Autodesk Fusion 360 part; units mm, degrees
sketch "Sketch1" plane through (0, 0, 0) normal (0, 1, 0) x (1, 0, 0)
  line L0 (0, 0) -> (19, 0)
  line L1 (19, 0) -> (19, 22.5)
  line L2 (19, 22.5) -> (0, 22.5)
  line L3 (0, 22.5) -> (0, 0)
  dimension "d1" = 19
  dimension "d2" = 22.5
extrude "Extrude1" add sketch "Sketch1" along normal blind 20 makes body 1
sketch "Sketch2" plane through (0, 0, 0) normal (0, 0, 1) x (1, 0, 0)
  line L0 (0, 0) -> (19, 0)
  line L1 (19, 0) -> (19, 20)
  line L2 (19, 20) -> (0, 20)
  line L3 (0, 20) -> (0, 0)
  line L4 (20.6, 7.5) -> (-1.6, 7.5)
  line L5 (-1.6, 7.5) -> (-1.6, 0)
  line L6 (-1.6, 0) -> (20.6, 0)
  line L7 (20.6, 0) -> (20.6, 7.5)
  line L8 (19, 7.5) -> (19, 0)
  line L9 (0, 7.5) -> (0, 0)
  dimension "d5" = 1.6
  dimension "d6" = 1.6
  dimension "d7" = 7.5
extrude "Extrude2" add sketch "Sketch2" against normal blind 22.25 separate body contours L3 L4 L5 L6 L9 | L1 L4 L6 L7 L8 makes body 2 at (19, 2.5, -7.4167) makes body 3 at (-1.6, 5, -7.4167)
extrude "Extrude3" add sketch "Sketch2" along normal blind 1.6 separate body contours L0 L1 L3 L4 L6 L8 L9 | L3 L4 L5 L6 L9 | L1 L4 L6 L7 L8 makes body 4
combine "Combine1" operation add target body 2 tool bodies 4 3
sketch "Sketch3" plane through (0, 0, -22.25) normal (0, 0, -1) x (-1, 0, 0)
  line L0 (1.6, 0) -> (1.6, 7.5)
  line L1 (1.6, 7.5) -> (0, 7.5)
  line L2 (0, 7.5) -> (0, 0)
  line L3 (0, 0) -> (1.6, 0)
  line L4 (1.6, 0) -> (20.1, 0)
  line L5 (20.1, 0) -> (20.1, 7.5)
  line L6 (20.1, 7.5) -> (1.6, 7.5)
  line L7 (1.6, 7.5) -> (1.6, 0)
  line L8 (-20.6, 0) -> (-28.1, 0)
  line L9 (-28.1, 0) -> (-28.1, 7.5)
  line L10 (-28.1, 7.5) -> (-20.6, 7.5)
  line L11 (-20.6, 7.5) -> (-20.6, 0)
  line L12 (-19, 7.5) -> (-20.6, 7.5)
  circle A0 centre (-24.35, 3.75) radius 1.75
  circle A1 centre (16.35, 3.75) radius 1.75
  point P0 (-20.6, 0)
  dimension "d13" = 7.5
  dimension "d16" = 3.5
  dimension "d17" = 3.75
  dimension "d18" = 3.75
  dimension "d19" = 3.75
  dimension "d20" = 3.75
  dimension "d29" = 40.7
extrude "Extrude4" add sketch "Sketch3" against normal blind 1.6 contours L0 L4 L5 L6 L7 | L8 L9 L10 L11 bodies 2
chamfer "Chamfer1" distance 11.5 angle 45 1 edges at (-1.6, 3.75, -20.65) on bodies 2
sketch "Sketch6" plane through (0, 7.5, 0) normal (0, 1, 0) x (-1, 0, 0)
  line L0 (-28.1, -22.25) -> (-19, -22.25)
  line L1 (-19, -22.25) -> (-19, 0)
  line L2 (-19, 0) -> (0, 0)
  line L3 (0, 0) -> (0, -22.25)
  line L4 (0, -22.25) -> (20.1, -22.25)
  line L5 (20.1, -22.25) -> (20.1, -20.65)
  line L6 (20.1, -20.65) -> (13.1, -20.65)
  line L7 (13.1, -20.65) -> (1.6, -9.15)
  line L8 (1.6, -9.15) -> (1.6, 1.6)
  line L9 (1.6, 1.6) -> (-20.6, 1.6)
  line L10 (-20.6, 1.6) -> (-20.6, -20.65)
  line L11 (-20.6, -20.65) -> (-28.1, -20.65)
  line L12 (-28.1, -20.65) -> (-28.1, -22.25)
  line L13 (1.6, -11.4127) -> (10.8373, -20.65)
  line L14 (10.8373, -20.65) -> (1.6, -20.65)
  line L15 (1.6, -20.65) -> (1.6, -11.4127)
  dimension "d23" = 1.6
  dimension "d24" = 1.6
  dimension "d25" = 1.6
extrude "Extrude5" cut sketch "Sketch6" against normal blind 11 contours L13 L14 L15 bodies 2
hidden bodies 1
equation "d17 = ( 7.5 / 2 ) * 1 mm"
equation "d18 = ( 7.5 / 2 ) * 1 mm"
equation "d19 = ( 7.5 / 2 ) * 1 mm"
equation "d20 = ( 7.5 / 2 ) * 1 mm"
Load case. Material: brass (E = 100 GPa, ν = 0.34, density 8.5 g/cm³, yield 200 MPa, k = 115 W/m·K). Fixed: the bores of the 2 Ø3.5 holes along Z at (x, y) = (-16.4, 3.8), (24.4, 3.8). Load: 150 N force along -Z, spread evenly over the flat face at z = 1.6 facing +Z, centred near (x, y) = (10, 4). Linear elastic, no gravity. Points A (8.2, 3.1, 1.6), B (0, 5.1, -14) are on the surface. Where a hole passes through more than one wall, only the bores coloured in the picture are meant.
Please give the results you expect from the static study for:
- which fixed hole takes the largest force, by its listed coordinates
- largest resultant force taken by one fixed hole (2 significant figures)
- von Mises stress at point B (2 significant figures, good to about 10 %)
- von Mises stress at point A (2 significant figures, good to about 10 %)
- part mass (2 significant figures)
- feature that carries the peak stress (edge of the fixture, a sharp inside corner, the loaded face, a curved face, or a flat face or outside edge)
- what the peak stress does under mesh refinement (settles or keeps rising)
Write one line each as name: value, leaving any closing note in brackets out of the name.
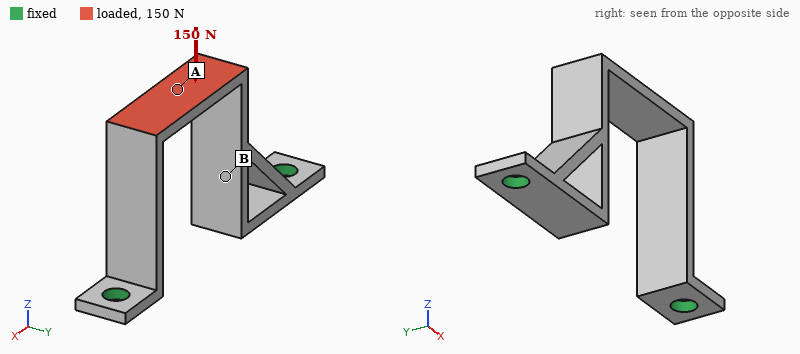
which fixed hole takes the largest force, by its listed coordinates: (24.4, 3.8)
largest resultant force taken by one fixed hole: 91 N
von Mises stress at point B: 13 MPa
von Mises stress at point A: 51 MPa
part mass: 11 g
feature that carries the peak stress: edge of the fixture
what the peak stress does under mesh refinement: keeps rising
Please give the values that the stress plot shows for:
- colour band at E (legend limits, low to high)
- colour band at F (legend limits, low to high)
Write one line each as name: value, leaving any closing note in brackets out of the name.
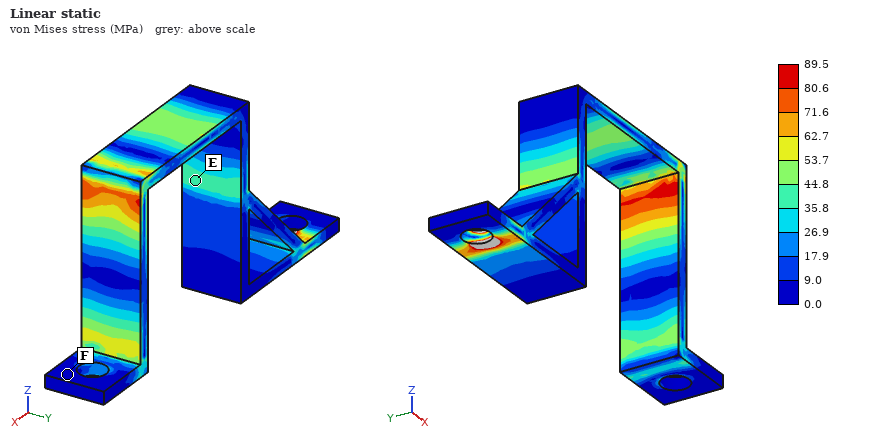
colour band at E: 35.8 to 44.8 MPa
colour band at F: 0.0 to 9.0 MPa
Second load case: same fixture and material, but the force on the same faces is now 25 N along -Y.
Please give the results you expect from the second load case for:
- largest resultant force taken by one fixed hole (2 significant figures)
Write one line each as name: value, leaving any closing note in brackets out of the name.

largest resultant force taken by one fixed hole: 13 N
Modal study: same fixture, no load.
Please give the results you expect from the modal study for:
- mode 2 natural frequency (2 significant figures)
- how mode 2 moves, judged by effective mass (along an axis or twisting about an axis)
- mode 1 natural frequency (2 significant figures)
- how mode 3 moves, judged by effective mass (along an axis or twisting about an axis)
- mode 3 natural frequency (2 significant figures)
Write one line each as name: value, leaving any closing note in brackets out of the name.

mode 2 natural frequency: 2000 Hz
how mode 2 moves, judged by effective mass: along Y
mode 1 natural frequency: 1700 Hz
how mode 3 moves, judged by effective mass: twisting about Z
mode 3 natural frequency: 3600 Hz
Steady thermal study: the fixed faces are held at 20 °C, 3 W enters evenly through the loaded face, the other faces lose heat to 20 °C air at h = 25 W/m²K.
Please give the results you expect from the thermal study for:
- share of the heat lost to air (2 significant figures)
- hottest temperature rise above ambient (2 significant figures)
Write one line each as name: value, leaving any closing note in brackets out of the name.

share of the heat lost to air: 16 %
hottest temperature rise above ambient: 28 K
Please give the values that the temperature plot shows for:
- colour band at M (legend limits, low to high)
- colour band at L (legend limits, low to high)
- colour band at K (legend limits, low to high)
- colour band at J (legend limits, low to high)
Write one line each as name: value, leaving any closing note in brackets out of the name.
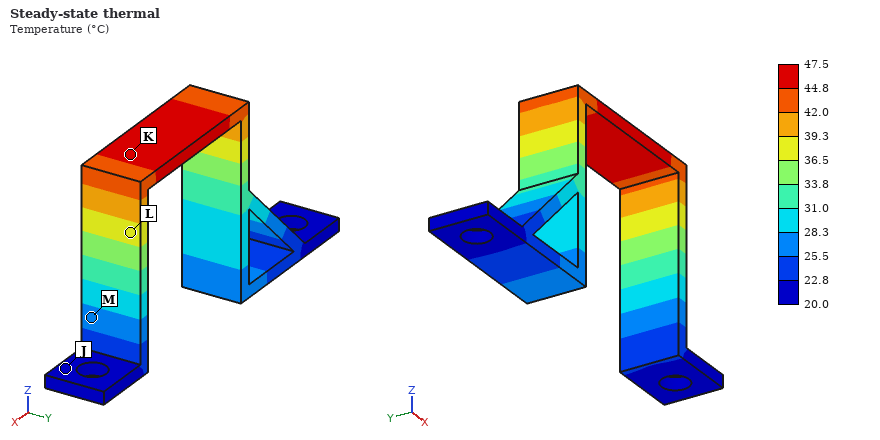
colour band at M: 25.5 to 28.3 °C
colour band at L: 36.5 to 39.3 °C
colour band at K: 44.8 to 47.5 °C
colour band at J: 20.0 to 22.8 °C
